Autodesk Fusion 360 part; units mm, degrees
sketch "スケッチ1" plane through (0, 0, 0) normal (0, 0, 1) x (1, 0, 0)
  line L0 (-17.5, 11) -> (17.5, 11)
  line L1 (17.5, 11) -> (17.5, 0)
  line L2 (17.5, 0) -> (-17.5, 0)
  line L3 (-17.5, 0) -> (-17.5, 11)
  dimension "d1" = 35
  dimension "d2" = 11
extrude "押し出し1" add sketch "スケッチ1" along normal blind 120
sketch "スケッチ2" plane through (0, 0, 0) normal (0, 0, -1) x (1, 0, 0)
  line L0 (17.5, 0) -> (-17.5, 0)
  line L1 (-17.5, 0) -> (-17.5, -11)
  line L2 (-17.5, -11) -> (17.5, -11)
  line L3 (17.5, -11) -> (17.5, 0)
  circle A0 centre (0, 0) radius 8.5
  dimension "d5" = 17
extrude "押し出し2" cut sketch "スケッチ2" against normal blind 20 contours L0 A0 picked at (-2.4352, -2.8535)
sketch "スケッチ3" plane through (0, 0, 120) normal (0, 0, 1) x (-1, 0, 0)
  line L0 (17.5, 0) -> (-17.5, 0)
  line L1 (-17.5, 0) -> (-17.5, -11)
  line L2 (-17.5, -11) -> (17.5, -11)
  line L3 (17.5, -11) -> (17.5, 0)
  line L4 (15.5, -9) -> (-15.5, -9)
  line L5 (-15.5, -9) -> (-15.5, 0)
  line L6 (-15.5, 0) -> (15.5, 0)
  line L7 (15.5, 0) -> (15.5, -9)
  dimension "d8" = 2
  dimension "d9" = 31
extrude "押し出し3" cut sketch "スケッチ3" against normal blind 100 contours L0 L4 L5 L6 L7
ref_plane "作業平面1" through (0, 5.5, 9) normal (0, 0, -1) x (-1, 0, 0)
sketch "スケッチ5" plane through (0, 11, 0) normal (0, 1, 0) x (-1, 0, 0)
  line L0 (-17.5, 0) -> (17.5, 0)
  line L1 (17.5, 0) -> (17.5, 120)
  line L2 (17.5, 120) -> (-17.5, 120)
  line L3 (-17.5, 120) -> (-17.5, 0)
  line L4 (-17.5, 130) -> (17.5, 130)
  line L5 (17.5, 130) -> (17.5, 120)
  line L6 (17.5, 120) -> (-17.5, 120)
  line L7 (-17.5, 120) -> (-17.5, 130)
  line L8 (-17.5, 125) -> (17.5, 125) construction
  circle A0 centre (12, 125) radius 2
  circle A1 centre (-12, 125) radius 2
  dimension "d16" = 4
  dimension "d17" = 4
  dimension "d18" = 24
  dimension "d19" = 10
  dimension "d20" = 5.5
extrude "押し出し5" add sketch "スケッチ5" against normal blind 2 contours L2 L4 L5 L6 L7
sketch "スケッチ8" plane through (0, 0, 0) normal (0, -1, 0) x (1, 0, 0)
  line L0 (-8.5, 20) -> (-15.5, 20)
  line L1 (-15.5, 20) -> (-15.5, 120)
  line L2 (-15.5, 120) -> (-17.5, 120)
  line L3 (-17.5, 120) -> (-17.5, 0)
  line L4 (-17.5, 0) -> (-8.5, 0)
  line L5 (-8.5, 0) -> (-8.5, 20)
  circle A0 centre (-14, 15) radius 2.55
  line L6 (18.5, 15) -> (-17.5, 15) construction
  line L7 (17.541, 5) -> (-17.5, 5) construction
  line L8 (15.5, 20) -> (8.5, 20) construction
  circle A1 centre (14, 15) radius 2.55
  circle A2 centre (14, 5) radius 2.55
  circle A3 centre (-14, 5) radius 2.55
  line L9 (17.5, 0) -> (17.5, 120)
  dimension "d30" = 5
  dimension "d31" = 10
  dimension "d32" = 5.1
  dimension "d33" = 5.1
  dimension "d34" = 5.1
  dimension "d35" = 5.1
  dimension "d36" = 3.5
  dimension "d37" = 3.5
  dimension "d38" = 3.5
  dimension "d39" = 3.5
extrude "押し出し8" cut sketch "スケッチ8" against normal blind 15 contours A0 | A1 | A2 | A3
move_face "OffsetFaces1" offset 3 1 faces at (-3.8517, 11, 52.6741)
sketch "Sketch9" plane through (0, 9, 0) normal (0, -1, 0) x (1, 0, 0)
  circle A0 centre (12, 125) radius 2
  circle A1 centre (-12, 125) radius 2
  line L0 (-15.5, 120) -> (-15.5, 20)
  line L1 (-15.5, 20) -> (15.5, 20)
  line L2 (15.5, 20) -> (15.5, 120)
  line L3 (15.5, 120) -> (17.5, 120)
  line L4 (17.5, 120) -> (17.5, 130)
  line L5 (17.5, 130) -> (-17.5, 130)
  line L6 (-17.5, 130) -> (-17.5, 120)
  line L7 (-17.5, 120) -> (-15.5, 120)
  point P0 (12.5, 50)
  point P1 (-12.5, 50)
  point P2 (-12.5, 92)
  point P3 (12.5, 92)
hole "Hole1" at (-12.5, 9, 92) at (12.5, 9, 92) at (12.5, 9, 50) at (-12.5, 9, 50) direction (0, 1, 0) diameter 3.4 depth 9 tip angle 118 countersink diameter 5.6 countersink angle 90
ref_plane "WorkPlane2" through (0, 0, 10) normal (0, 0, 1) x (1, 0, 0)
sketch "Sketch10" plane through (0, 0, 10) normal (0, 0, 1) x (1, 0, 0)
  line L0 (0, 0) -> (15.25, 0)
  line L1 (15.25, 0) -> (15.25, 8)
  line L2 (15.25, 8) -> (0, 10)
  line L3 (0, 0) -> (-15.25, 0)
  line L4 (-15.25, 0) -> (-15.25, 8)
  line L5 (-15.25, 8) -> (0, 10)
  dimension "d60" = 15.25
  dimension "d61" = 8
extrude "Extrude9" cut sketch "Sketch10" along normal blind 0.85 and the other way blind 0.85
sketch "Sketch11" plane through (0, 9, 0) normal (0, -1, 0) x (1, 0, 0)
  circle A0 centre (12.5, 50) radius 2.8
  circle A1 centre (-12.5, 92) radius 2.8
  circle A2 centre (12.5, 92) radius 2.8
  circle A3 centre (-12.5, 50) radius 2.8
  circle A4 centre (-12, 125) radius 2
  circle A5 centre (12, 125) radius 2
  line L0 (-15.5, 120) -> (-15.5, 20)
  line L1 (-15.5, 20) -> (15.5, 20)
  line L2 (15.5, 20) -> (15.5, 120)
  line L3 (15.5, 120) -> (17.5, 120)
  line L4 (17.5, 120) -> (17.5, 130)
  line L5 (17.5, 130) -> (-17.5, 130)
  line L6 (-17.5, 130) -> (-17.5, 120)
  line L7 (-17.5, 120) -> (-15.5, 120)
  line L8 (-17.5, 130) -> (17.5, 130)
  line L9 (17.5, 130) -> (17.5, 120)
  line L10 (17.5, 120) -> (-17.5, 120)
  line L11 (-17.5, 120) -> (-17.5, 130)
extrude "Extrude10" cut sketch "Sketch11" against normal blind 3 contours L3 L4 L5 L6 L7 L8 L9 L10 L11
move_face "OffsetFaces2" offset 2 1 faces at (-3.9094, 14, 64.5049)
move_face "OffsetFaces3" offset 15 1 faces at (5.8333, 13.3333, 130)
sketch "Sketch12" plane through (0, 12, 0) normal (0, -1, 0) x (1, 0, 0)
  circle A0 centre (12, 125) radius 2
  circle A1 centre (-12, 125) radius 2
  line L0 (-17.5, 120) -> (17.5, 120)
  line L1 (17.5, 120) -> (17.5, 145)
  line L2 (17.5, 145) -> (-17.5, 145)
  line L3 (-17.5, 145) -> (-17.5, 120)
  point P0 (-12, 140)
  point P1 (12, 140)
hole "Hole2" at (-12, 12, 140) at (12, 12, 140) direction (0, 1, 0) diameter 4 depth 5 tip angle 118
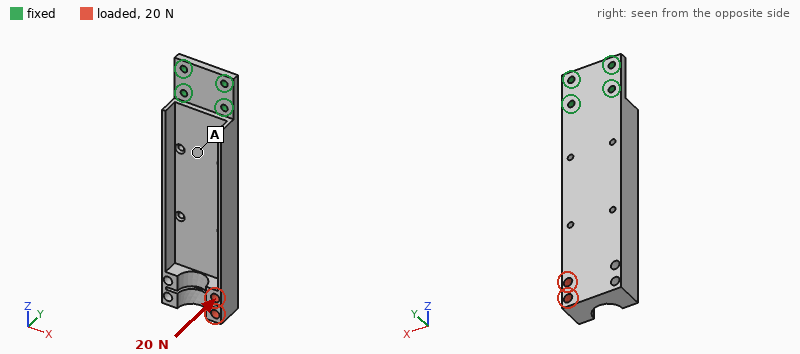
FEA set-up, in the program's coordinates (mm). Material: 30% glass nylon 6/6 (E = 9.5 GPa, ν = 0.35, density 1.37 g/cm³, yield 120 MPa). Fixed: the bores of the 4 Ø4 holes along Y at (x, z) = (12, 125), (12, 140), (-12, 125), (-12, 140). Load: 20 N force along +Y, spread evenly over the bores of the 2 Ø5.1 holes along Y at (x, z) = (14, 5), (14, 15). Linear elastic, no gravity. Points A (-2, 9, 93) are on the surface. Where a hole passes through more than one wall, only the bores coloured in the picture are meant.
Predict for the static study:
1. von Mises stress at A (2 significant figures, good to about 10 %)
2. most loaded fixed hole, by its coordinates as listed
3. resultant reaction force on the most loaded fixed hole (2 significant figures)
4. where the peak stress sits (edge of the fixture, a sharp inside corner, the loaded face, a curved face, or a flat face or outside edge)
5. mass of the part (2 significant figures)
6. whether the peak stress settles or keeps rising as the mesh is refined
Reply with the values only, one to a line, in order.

2.0 MPa
(12, 125)
46 N
edge of the fixture
53 g
keeps rising
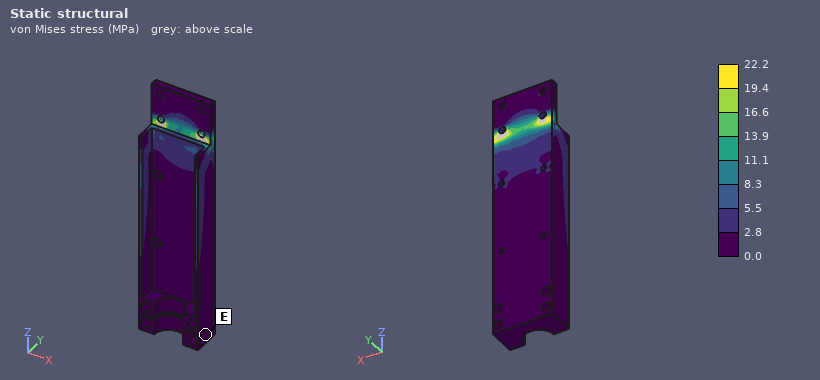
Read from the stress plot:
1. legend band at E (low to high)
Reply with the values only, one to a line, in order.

0.0 to 2.8 MPa
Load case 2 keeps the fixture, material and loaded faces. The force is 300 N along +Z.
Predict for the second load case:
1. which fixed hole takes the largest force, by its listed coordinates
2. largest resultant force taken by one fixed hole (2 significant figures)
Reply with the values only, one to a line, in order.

(12, 125)
280 N
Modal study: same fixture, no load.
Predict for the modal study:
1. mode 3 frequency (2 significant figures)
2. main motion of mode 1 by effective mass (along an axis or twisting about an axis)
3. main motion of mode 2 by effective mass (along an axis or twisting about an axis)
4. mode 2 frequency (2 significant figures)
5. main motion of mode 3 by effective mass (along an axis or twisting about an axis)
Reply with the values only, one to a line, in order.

970 Hz
along Y
along X
730 Hz
twisting about Z
